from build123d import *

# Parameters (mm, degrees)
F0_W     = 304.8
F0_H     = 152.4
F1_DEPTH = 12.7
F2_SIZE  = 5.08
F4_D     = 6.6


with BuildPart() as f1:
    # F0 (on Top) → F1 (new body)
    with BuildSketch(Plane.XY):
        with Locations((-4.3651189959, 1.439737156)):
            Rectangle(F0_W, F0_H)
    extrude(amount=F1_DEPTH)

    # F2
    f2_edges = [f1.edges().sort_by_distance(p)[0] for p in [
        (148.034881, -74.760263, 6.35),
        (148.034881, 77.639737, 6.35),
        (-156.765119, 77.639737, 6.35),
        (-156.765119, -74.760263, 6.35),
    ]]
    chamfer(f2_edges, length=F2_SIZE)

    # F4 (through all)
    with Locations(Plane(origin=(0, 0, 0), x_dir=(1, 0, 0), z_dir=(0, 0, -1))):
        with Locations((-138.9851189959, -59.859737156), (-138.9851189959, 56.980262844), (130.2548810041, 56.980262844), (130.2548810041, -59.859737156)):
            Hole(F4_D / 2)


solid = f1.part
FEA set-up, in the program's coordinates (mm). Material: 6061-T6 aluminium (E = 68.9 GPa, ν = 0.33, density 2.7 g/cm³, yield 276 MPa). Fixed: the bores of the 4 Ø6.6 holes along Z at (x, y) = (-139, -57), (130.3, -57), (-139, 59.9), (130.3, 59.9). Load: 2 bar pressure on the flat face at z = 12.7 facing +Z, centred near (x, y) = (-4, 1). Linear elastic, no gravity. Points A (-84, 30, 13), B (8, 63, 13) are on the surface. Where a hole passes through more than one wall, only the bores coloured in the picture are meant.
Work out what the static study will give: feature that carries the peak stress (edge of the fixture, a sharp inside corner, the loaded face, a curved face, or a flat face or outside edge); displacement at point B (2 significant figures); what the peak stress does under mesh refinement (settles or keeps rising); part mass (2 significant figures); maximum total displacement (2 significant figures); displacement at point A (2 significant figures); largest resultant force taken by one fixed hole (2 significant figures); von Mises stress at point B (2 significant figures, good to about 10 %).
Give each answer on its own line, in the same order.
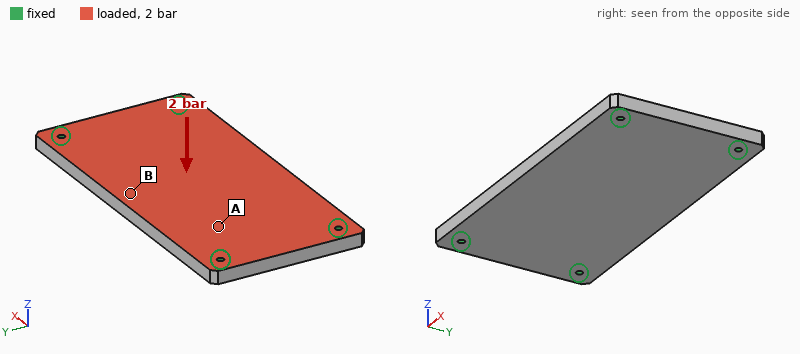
edge of the fixture
0.33 mm
keeps rising
1.6 kg
0.34 mm
0.17 mm
2.3 kN
27 MPa
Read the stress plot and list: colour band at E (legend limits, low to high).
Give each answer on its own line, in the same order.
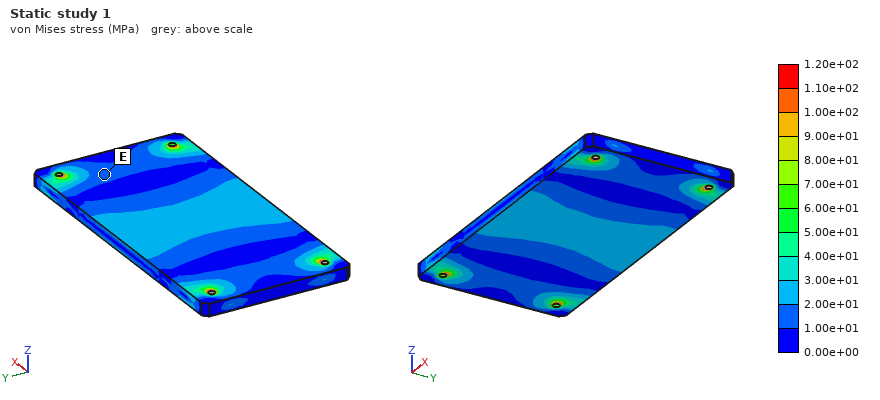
1.00e+01 to 2.00e+01 MPa
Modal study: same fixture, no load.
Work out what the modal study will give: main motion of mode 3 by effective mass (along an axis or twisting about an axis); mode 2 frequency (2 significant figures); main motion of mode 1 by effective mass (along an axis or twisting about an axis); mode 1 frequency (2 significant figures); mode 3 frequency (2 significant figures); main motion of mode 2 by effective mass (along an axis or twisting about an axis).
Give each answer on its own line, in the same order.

twisting about Y
1300 Hz
along Z
760 Hz
2100 Hz
twisting about X
